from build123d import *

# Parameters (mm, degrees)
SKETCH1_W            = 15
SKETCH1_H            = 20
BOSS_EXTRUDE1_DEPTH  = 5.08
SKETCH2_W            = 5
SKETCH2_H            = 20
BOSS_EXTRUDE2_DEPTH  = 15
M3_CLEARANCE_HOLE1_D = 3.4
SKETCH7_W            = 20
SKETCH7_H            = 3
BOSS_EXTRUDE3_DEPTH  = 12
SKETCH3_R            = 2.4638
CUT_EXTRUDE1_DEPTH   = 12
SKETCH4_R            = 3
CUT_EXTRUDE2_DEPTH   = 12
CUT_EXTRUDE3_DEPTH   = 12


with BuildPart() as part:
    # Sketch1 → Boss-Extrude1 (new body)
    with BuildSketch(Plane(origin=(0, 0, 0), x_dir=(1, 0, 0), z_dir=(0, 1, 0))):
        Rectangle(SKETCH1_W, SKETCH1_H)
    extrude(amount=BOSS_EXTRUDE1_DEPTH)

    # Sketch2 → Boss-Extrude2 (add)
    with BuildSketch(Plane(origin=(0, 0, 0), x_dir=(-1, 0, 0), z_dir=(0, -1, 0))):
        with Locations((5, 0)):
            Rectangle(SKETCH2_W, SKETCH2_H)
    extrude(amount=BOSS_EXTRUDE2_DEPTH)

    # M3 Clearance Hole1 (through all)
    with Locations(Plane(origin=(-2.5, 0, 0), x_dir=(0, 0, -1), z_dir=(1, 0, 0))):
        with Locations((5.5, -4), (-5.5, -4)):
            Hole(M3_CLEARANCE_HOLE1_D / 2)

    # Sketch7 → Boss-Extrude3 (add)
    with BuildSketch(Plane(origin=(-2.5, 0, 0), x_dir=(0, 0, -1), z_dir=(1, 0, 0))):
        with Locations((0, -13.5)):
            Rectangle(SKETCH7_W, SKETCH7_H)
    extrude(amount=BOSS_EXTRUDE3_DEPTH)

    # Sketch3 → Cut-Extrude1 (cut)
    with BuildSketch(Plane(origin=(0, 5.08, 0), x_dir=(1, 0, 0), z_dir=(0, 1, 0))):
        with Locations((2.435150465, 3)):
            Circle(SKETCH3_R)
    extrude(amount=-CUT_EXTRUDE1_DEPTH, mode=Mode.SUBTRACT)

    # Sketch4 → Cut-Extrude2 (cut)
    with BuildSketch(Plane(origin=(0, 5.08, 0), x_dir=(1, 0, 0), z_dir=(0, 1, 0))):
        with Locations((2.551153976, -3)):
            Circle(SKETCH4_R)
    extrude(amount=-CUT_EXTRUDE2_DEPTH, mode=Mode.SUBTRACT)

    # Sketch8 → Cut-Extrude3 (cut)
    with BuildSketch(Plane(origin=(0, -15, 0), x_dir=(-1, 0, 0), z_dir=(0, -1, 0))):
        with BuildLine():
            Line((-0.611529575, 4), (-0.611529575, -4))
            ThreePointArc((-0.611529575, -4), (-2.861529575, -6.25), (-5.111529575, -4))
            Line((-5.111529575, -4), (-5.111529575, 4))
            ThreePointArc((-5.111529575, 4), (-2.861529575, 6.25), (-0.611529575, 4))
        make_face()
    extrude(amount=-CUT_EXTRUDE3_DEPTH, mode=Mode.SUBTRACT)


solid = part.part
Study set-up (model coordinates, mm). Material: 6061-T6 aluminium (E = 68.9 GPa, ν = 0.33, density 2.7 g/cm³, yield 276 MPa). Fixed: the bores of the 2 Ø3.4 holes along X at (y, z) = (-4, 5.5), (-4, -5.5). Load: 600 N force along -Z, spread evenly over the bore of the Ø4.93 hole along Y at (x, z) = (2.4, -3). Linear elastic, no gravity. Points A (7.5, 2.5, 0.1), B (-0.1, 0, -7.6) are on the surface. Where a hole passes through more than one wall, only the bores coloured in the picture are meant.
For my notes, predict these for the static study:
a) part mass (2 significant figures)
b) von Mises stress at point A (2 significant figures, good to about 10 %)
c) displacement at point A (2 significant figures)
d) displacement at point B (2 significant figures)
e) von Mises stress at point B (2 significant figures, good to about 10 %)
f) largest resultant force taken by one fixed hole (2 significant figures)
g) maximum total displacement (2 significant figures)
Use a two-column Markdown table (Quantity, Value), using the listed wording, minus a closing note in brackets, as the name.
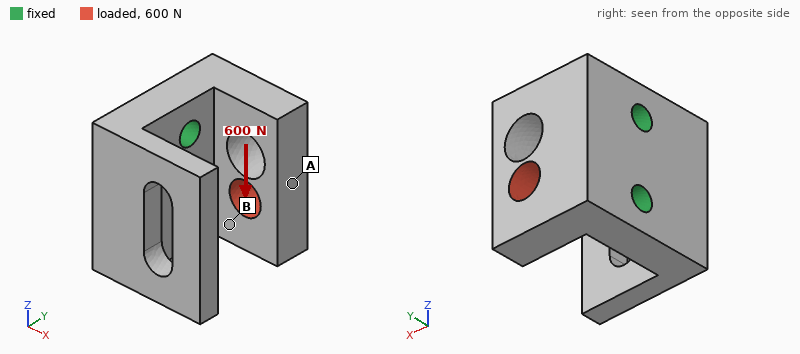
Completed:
| Quantity | Value |
|---|---|
| part mass | 8.8 g |
| von Mises stress at point A | 9.9 MPa |
| displacement at point A | 13 µm |
| displacement at point B | 6.4 µm |
| von Mises stress at point B | 21 MPa |
| largest resultant force taken by one fixed hole | 500 N |
| maximum total displacement | 17 µm |
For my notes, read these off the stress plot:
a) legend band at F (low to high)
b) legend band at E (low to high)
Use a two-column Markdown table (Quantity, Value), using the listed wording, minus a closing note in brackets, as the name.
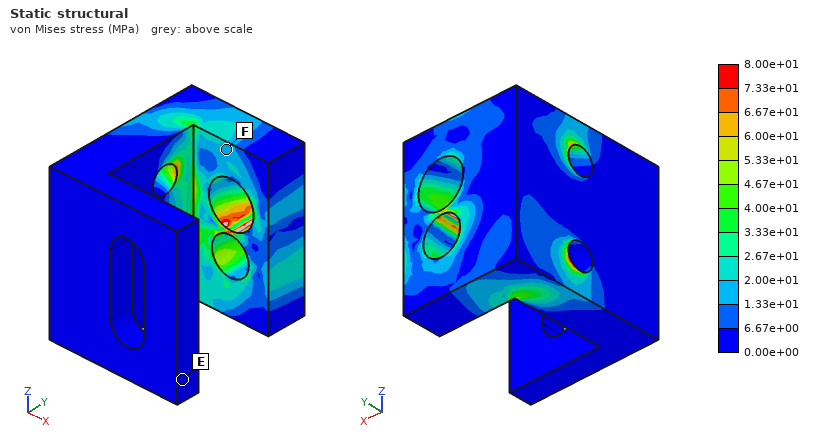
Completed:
| Quantity | Value |
|---|---|
| legend band at F | 1.33e+01 to 2.00e+01 MPa |
| legend band at E | 0.00e+00 to 6.67e+00 MPa |
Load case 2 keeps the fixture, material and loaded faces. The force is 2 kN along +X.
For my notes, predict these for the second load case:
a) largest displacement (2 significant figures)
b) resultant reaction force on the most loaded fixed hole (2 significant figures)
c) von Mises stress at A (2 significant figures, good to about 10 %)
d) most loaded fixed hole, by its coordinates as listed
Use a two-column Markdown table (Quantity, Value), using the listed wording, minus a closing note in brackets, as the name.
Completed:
| Quantity | Value |
|---|---|
| largest displacement | 52 µm |
| resultant reaction force on the most loaded fixed hole | 1.4 kN |
| von Mises stress at A | 37 MPa |
| most loaded fixed hole, by its coordinates as listed | (-4, -5.5) |
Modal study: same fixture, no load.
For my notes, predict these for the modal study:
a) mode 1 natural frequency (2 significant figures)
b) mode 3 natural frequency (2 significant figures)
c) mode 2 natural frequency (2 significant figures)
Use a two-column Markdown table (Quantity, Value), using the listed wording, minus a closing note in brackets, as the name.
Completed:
| Quantity | Value |
|---|---|
| mode 1 natural frequency | 9000 Hz |
| mode 3 natural frequency | 16 kHz |
| mode 2 natural frequency | 16 kHz |
